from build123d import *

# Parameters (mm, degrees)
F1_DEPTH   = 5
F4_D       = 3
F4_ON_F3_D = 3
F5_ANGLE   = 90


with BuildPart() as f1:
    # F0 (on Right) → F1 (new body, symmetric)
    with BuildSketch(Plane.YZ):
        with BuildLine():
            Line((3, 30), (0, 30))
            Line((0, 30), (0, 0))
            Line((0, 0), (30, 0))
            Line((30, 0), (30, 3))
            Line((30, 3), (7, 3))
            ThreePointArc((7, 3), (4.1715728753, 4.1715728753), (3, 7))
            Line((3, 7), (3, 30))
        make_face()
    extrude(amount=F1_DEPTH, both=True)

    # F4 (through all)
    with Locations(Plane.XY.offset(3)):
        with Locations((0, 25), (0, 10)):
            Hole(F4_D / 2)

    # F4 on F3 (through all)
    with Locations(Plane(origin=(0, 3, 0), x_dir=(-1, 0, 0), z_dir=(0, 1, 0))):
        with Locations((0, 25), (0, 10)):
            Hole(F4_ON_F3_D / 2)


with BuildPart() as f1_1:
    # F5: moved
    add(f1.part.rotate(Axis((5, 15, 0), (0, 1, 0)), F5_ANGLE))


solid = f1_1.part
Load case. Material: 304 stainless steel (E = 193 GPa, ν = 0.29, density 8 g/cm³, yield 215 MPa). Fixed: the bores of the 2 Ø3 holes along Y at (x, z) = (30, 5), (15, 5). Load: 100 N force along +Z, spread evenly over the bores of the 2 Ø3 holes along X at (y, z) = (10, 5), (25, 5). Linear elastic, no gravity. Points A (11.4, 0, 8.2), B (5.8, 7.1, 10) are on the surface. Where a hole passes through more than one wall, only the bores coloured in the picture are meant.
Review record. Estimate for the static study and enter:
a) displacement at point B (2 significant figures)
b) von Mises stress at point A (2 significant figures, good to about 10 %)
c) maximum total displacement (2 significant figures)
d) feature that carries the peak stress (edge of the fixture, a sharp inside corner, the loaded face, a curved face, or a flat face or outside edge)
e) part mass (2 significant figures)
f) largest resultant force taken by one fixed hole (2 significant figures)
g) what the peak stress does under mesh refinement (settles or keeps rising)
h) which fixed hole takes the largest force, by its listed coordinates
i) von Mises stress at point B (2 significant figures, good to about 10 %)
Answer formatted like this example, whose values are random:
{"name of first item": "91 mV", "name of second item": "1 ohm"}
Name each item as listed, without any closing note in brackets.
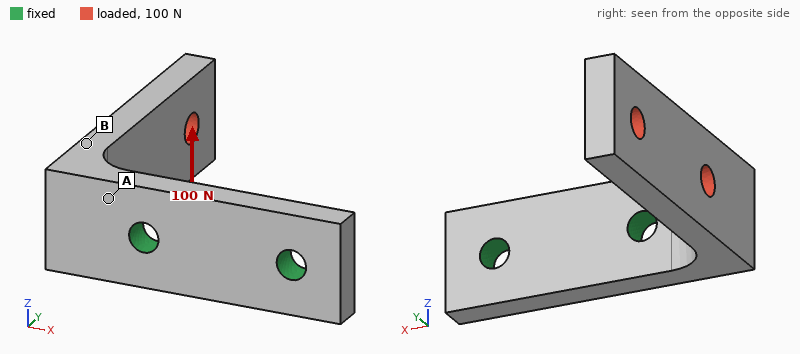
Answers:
{"displacement at point B": "11 µm", "von Mises stress at point A": "47 MPa", "maximum total displacement": "44 µm", "feature that carries the peak stress": "edge of the fixture", "part mass": "13 g", "largest resultant force taken by one fixed hole": "130 N", "what the peak stress does under mesh refinement": "keeps rising", "which fixed hole takes the largest force, by its listed coordinates": "(15, 5)", "von Mises stress at point B": "20 MPa"}
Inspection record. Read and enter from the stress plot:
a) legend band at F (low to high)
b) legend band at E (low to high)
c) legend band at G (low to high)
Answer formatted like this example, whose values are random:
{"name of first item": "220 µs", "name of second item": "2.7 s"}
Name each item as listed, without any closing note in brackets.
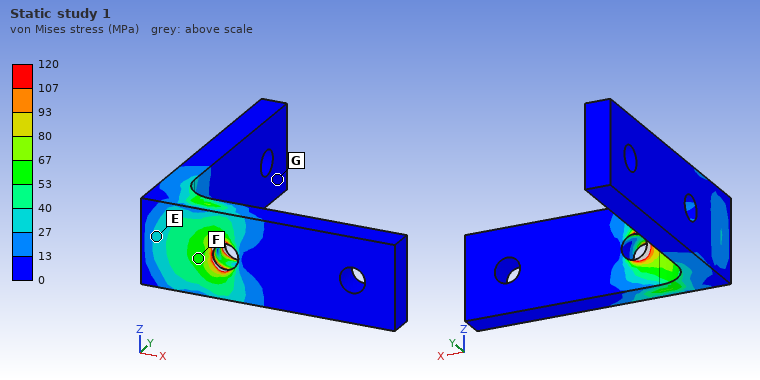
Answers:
{"legend band at F": "53 to 67 MPa", "legend band at E": "27 to 40 MPa", "legend band at G": "0 to 13 MPa"}
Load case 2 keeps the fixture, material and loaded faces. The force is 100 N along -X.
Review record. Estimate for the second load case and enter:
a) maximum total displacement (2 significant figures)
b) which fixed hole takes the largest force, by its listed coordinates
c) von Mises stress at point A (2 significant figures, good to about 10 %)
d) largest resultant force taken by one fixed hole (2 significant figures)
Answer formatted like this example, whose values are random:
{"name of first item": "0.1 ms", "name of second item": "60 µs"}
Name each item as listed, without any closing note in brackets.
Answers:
{"maximum total displacement": "0.12 mm", "which fixed hole takes the largest force, by its listed coordinates": "(15, 5)", "von Mises stress at point A": "86 MPa", "largest resultant force taken by one fixed hole": "94 N"}
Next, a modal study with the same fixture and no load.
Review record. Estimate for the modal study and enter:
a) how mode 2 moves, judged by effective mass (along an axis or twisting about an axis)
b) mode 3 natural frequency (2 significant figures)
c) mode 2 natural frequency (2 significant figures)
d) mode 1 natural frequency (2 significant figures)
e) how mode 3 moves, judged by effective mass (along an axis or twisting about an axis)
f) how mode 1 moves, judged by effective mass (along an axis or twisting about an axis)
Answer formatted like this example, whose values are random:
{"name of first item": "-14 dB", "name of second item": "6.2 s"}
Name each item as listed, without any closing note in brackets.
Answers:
{"how mode 2 moves, judged by effective mass": "along Z", "mode 3 natural frequency": "10 kHz", "mode 2 natural frequency": "3900 Hz", "mode 1 natural frequency": "2400 Hz", "how mode 3 moves, judged by effective mass": "along Y", "how mode 1 moves, judged by effective mass": "along X"}
